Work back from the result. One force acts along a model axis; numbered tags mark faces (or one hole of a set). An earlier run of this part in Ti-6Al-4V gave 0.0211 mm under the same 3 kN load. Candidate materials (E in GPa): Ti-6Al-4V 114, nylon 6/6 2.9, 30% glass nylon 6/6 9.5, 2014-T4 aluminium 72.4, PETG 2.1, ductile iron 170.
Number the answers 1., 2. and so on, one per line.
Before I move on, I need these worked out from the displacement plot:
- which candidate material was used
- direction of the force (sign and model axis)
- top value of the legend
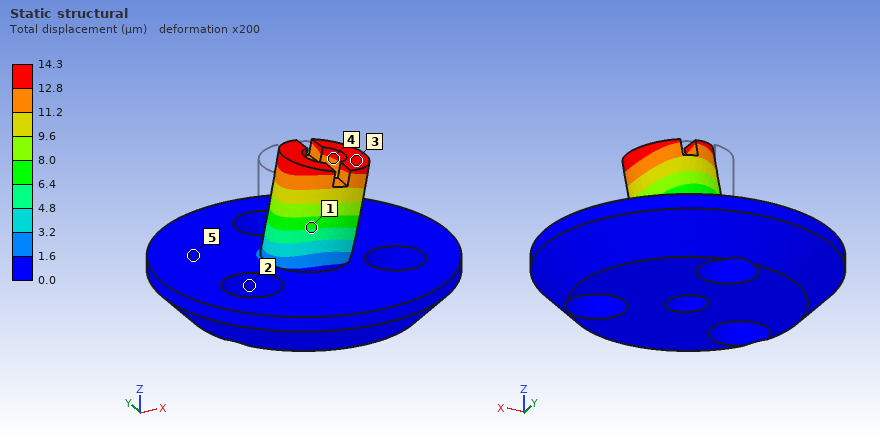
1. ductile iron
2. +X
3. 14.3 µm
